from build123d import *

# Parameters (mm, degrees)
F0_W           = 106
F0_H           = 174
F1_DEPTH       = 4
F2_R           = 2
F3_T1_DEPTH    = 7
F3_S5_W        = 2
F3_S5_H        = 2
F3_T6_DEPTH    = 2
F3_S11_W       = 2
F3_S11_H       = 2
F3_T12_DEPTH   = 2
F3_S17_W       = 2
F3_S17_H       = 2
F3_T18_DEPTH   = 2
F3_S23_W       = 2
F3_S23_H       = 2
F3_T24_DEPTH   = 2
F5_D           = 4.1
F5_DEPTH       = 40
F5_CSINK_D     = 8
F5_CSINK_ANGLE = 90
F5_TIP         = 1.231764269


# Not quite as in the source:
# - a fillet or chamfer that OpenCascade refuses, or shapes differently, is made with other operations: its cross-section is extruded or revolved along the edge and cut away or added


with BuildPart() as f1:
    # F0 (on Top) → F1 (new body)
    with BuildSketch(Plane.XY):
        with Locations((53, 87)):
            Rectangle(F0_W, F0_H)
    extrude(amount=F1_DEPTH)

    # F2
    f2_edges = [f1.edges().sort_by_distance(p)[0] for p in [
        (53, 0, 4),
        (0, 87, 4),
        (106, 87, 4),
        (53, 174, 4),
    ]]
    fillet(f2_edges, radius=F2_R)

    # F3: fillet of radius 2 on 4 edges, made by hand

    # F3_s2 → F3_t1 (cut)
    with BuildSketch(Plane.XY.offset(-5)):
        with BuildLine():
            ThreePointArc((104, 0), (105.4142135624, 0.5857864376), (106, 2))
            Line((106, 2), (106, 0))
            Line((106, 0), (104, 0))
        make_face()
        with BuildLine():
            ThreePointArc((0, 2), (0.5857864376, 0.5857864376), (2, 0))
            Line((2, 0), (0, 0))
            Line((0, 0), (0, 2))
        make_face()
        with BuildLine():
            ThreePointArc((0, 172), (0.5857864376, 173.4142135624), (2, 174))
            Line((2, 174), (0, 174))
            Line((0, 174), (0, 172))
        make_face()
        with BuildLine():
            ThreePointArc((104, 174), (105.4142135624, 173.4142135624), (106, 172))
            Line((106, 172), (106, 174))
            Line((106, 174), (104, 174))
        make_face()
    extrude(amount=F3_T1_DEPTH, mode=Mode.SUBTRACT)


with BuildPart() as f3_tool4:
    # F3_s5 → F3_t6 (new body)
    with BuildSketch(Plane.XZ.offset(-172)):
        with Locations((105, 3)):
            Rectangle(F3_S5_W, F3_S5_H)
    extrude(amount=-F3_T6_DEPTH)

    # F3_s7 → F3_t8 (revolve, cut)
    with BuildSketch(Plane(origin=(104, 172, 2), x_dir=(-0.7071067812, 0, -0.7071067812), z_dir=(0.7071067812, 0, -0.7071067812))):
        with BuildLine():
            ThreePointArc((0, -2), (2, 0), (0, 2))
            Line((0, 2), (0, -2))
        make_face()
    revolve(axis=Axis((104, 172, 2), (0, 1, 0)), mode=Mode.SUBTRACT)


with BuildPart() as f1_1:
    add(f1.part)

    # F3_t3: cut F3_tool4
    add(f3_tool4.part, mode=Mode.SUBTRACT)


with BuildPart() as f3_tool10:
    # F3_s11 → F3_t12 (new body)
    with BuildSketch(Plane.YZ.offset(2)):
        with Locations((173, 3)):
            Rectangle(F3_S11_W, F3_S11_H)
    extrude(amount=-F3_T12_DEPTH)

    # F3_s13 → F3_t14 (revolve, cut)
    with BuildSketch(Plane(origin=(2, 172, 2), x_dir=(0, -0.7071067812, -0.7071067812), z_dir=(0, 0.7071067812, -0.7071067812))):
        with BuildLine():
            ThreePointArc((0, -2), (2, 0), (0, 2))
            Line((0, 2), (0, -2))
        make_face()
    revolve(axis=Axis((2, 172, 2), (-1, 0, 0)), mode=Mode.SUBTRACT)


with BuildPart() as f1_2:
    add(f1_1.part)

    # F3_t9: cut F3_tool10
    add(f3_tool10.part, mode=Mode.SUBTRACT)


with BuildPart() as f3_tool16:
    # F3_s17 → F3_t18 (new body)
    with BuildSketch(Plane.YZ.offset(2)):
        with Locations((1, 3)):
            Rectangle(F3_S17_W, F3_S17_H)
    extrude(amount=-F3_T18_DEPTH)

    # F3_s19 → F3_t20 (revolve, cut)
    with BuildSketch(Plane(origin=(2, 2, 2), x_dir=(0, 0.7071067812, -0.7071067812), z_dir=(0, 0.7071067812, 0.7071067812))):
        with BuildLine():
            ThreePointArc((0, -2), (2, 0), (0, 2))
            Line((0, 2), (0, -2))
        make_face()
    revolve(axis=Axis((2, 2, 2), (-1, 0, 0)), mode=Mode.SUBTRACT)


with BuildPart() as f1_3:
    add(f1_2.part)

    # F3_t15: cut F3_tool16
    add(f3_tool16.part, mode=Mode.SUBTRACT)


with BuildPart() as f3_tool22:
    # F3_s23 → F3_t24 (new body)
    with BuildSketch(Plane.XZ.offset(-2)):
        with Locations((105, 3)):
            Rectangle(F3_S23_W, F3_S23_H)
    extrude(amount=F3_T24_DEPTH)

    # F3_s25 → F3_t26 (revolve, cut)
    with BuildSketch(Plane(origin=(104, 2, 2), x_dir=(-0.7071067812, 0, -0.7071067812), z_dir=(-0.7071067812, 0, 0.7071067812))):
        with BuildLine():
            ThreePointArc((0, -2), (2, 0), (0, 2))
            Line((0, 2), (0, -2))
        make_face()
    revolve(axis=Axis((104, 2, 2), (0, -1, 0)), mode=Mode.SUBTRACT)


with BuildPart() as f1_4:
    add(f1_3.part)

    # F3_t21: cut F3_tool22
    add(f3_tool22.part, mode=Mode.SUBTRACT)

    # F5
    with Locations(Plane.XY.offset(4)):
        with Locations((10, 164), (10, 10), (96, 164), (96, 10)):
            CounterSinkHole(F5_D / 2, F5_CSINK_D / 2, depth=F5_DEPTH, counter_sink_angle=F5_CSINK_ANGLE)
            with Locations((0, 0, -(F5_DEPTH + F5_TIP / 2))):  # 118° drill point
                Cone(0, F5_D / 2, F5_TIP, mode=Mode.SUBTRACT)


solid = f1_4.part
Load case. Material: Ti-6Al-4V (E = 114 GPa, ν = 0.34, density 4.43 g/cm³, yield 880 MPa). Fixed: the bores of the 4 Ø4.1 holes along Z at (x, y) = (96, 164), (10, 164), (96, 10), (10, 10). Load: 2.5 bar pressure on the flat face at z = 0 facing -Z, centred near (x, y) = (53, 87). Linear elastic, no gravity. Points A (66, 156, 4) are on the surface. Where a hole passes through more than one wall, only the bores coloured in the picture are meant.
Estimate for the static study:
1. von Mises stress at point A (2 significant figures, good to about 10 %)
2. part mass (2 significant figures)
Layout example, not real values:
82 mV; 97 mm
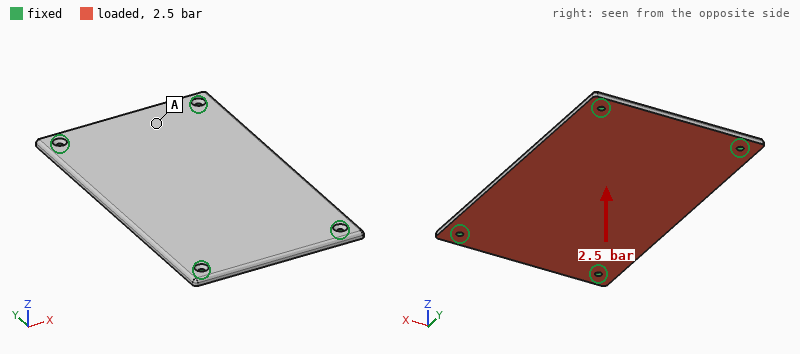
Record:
58 MPa; 320 g
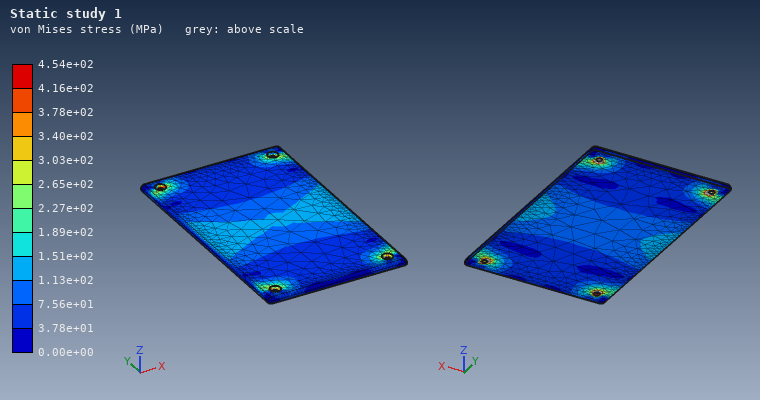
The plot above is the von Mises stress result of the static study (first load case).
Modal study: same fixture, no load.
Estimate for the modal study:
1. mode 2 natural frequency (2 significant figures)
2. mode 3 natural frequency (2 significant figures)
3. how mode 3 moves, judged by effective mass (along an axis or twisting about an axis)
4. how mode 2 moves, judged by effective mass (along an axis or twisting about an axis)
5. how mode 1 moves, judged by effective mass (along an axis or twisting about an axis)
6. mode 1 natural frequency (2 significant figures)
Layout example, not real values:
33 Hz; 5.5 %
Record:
1100 Hz; 1800 Hz; twisting about X; twisting about Y; along Z; 660 Hz
